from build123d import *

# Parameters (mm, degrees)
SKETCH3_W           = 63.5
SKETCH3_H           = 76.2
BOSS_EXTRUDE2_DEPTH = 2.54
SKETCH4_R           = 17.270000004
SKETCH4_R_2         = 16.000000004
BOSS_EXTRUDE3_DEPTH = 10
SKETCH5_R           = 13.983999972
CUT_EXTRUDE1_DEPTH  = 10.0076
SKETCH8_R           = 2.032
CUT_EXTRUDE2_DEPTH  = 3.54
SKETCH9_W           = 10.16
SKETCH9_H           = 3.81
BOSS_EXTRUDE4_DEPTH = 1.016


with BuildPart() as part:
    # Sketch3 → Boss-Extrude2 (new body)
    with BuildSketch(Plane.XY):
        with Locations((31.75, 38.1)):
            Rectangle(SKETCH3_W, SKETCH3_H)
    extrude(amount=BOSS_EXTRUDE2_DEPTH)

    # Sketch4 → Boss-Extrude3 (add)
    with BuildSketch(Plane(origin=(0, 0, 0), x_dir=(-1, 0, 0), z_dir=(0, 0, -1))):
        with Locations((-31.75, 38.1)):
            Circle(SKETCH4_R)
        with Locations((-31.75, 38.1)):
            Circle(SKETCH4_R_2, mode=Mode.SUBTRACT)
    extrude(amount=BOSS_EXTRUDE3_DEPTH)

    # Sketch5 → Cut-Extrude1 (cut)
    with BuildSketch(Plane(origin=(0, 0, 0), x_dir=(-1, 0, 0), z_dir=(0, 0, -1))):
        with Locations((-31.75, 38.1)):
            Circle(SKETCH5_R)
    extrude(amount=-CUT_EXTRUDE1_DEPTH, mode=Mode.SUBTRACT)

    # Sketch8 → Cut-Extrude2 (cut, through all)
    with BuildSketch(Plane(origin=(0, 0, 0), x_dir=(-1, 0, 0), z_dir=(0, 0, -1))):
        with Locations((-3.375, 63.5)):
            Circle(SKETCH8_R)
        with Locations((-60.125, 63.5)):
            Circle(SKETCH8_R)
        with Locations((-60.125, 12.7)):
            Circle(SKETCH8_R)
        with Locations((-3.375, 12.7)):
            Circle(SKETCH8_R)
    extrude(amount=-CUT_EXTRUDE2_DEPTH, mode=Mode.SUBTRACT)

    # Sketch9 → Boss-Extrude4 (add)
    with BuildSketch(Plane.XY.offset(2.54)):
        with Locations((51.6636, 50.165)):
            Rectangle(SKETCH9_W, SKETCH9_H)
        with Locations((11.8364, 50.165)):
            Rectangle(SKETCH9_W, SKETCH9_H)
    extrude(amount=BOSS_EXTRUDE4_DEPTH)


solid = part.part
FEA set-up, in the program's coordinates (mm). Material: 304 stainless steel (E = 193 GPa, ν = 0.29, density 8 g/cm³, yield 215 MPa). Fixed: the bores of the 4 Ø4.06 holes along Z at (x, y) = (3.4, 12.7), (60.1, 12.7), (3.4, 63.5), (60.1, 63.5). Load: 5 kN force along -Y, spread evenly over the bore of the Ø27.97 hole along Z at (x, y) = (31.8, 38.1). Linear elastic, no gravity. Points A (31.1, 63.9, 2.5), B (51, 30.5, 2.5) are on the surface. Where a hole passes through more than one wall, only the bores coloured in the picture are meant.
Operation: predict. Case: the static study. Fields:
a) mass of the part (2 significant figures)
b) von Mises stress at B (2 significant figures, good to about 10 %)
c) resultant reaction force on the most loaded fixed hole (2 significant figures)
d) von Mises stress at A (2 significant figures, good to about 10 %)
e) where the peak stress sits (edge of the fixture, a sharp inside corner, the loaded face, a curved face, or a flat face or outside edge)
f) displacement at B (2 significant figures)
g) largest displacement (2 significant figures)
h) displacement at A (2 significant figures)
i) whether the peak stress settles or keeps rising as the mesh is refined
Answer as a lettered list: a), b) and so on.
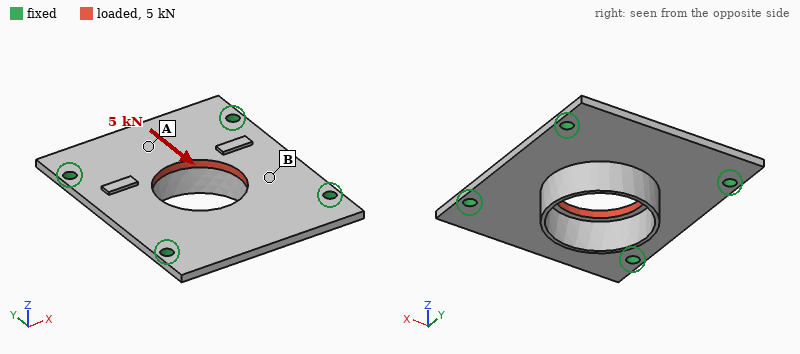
a) 96 g
b) 29 MPa
c) 1.3 kN
d) 11 MPa
e) edge of the fixture
f) 3.6 µm
g) 7.1 µm
h) 6.1 µm
i) keeps rising
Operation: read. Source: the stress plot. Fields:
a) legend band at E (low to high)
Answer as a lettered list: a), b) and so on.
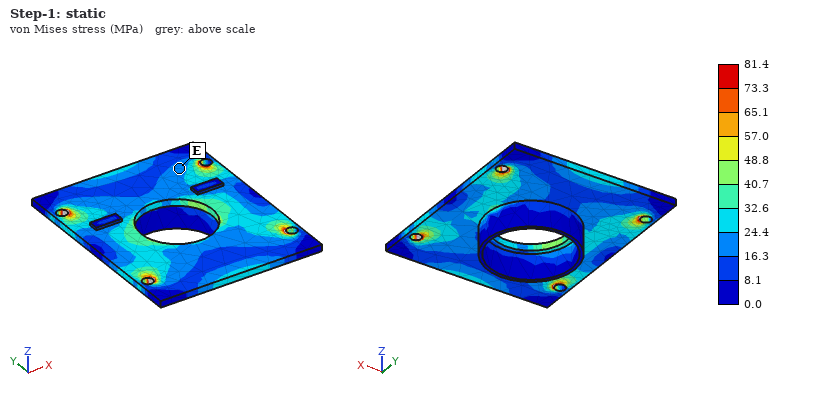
a) 16.3 to 24.4 MPa
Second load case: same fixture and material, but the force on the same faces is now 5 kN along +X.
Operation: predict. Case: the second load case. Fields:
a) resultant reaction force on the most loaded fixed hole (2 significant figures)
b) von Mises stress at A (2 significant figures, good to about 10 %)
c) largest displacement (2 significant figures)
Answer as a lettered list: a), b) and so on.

a) 1.4 kN
b) 16 MPa
c) 6.9 µm
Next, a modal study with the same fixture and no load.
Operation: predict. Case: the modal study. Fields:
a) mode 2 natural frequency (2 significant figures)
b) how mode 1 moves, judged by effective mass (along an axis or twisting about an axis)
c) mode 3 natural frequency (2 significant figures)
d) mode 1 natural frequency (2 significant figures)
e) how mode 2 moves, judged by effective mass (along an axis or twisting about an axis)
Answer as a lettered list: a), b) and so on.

a) 4100 Hz
b) along Z
c) 4600 Hz
d) 3500 Hz
e) twisting about X
